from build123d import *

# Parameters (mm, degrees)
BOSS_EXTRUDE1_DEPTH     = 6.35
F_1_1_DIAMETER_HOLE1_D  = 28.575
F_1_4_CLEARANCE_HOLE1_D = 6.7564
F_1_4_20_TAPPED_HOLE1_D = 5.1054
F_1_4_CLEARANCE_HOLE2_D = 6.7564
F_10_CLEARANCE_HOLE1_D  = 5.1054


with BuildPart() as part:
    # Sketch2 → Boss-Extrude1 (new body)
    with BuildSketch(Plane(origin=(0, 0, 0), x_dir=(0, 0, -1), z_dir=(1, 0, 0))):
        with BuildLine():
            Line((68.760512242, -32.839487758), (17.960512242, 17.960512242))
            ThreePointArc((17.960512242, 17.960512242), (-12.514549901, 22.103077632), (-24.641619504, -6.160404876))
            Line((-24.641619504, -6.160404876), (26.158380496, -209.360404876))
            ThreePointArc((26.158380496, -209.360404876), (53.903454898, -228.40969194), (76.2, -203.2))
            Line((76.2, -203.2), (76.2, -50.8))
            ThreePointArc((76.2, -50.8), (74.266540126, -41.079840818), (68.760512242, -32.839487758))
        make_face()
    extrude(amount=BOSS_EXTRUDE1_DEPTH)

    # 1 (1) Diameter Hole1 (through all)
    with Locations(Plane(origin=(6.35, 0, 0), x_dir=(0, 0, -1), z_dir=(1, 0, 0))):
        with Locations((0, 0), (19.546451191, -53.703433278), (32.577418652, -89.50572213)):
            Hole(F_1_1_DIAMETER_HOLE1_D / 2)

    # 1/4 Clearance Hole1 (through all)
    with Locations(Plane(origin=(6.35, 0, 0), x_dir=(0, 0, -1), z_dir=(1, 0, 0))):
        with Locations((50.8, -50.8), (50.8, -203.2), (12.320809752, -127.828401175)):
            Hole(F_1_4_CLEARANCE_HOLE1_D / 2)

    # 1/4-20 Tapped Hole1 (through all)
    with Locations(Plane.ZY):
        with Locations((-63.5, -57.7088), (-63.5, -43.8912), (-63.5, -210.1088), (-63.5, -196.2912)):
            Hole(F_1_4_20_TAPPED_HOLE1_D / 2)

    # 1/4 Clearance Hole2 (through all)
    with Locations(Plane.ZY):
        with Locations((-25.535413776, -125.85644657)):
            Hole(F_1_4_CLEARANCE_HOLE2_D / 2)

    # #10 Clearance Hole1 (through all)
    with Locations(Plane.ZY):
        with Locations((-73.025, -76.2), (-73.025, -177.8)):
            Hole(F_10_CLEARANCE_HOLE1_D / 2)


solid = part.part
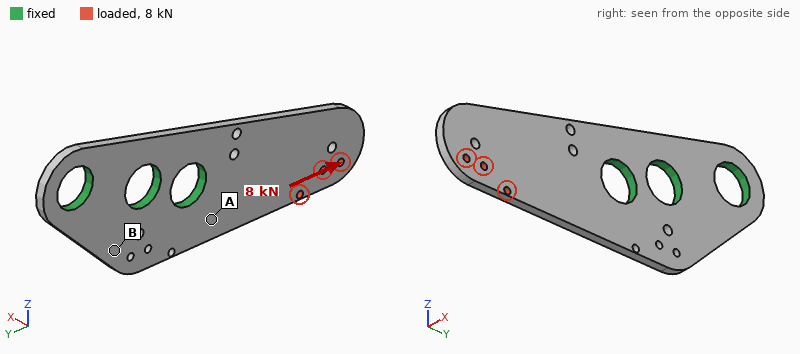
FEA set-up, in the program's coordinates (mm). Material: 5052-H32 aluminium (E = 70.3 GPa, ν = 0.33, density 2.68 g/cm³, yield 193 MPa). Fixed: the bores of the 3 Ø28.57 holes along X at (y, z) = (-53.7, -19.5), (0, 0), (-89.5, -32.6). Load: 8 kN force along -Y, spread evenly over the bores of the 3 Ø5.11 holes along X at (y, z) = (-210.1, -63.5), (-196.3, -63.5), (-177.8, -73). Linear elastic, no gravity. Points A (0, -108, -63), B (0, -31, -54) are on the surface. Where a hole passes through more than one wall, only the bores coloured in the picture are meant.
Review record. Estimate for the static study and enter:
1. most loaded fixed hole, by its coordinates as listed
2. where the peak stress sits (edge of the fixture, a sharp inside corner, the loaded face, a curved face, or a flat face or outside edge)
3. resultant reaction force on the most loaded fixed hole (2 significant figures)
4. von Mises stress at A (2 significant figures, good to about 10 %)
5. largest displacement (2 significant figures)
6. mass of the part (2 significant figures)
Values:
(-89.5, -32.6)
the loaded face
7.7 kN
38 MPa
0.21 mm
250 g
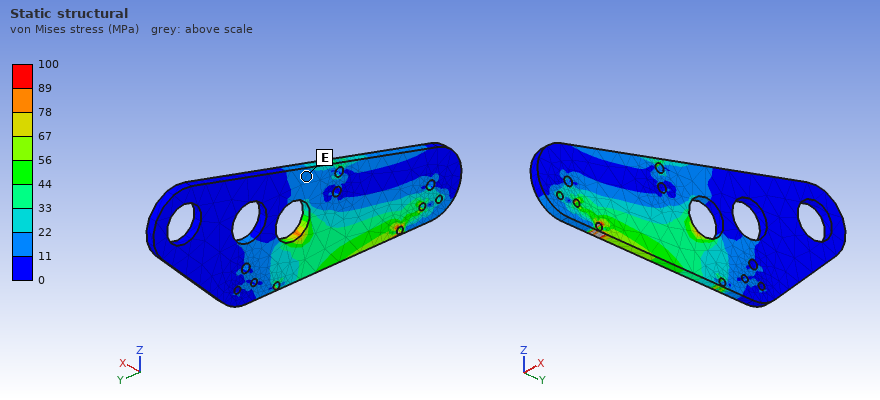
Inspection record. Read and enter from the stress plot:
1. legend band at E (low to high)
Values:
11 to 22 MPa
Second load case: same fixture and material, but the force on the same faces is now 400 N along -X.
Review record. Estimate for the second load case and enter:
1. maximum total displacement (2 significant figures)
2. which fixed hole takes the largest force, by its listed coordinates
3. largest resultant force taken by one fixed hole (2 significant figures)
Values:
1.9 mm
(-89.5, -32.6)
450 N
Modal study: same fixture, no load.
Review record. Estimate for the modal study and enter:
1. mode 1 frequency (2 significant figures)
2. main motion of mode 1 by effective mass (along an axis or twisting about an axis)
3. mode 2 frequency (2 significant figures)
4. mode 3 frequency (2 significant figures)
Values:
390 Hz
along X
1600 Hz
2100 Hz
